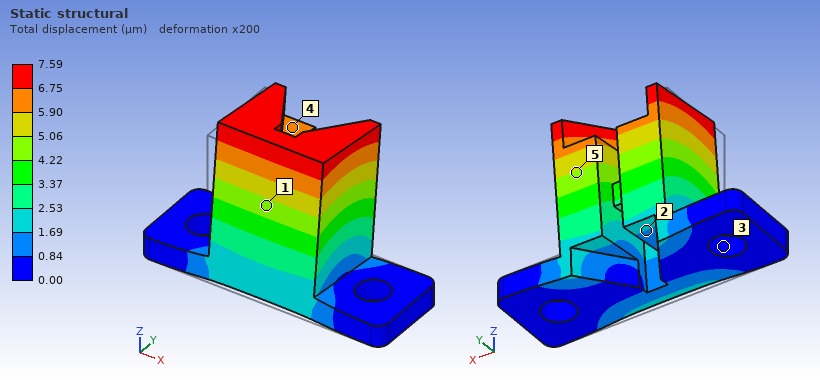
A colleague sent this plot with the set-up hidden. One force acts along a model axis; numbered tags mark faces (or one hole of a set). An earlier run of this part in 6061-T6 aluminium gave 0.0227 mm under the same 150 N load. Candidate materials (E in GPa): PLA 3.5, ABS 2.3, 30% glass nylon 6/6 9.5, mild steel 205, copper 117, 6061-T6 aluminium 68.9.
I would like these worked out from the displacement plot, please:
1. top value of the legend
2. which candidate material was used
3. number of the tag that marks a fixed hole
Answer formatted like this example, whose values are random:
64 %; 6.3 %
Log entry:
7.59 µm; mild steel; 3
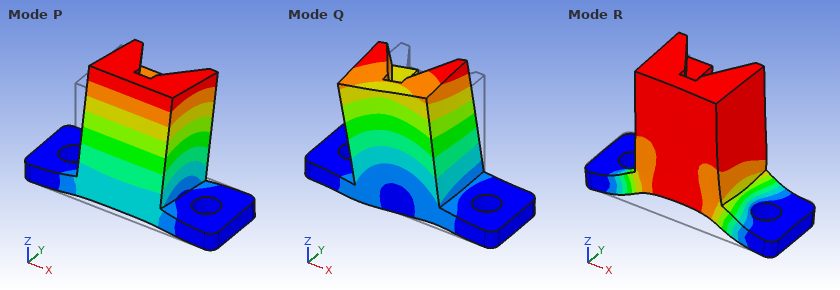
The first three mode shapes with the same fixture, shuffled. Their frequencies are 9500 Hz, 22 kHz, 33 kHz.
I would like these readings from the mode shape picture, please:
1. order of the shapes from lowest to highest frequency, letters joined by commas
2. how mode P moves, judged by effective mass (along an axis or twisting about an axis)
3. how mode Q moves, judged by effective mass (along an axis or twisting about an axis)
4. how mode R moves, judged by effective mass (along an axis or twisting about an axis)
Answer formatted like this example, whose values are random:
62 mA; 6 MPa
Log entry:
P, Q, R; along Y; along X; along Z
